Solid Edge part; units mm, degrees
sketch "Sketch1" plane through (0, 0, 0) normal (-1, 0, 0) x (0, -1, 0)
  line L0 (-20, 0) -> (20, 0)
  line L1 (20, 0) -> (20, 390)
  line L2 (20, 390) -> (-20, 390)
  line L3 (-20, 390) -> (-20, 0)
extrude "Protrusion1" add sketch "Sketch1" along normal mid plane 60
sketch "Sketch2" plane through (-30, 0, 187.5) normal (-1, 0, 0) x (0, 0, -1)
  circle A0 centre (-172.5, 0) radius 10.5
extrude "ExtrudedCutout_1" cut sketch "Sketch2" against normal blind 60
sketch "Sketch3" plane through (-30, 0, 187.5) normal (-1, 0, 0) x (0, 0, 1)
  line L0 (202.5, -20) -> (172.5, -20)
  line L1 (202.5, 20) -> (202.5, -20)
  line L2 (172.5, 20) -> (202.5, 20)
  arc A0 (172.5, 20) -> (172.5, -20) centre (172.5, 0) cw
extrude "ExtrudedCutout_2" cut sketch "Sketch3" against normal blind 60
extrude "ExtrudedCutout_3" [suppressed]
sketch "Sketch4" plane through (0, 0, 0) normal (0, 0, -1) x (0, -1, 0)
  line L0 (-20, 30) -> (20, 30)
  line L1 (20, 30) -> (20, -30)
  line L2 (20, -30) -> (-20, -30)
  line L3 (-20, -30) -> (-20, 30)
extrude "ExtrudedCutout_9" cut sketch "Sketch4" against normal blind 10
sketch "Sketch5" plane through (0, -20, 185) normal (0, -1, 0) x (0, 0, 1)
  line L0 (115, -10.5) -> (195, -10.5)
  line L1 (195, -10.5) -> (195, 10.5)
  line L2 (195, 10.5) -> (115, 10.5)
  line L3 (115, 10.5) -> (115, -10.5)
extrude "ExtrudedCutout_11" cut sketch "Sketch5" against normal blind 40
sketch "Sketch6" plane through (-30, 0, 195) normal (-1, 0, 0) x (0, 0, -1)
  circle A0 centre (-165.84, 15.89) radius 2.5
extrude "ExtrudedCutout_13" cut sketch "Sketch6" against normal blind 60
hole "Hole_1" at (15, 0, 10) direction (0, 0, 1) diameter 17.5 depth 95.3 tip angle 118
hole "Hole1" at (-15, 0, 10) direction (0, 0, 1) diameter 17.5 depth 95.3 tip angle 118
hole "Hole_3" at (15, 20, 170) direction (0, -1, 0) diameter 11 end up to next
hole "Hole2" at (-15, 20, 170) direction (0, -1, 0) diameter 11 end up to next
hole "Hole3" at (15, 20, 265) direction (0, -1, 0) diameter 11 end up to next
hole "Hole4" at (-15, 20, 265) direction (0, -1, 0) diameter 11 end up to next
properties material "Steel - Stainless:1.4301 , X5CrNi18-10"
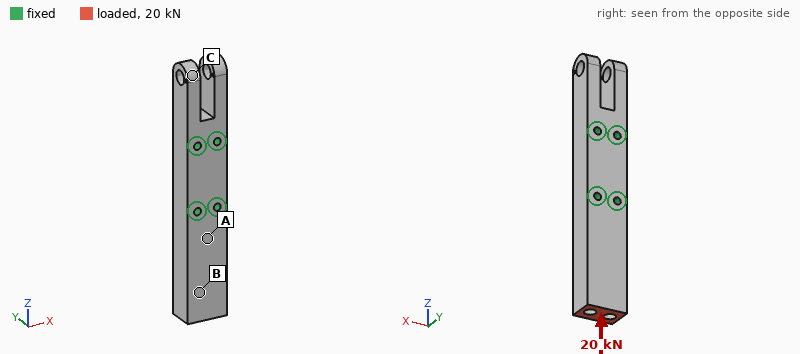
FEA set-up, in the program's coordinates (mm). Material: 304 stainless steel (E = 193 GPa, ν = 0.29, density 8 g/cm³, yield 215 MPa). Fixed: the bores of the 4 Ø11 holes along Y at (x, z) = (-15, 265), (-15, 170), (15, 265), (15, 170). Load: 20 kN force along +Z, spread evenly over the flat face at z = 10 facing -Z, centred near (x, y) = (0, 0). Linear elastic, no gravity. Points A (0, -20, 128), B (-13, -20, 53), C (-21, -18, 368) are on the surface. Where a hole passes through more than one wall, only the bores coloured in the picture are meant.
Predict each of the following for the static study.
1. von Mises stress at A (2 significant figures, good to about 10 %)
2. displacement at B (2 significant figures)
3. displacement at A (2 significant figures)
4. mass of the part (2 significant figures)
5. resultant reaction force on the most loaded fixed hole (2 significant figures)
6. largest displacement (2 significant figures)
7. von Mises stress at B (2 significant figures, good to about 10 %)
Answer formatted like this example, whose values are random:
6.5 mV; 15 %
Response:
8.8 MPa; 5.7 µm; 1.8 µm; 5.9 kg; 9.8 kN; 8.0 µm; 10 MPa
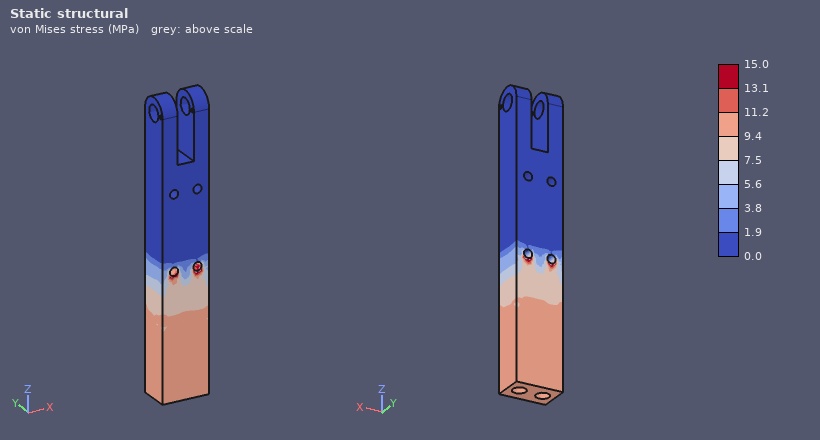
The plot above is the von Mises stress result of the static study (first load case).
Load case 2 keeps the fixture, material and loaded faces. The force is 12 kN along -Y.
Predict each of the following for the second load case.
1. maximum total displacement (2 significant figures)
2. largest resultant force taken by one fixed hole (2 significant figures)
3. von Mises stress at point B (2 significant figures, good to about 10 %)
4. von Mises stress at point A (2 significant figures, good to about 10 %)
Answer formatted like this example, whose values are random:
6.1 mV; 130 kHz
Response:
0.29 mm; 6.8 kN; 33 MPa; 88 MPa
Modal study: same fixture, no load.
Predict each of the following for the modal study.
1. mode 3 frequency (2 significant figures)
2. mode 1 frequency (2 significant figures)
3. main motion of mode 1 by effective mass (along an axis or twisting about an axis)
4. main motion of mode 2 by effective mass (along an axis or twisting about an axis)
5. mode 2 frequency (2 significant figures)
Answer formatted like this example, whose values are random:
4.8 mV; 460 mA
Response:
2200 Hz; 1300 Hz; along Y; along X; 1800 Hz
